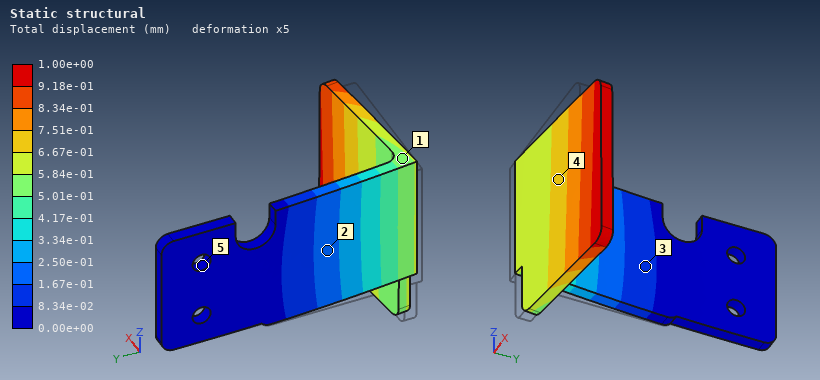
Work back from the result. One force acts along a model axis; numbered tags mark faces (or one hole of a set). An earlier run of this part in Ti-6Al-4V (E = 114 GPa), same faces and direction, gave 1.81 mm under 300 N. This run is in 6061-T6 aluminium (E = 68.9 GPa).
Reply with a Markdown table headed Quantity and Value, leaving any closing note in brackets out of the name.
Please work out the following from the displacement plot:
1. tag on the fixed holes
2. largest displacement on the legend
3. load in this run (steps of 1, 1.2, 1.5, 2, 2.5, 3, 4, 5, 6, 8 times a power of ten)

| Quantity | Value |
|---|---|
| tag on the fixed holes | 5 |
| largest displacement on the legend | 1.00e+00 mm |
| load in this run | 100 N |
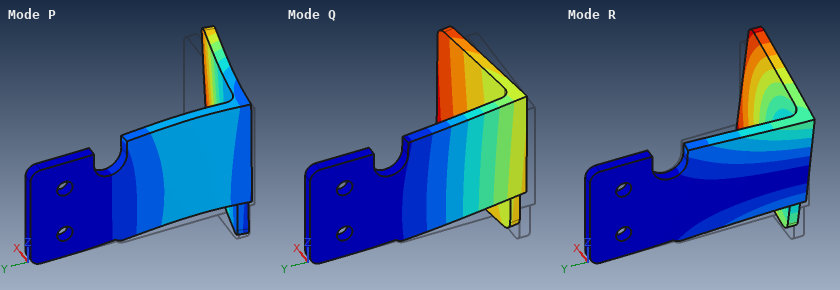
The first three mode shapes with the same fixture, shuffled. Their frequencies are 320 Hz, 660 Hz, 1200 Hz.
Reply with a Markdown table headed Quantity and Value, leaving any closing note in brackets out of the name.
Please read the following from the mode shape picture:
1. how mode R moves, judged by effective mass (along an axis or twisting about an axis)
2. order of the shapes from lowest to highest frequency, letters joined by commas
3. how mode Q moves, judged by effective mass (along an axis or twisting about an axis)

| Quantity | Value |
|---|---|
| how mode R moves, judged by effective mass | along Z |
| order of the shapes from lowest to highest frequency, letters joined by commas | Q, R, P |
| how mode Q moves, judged by effective mass | along X |
